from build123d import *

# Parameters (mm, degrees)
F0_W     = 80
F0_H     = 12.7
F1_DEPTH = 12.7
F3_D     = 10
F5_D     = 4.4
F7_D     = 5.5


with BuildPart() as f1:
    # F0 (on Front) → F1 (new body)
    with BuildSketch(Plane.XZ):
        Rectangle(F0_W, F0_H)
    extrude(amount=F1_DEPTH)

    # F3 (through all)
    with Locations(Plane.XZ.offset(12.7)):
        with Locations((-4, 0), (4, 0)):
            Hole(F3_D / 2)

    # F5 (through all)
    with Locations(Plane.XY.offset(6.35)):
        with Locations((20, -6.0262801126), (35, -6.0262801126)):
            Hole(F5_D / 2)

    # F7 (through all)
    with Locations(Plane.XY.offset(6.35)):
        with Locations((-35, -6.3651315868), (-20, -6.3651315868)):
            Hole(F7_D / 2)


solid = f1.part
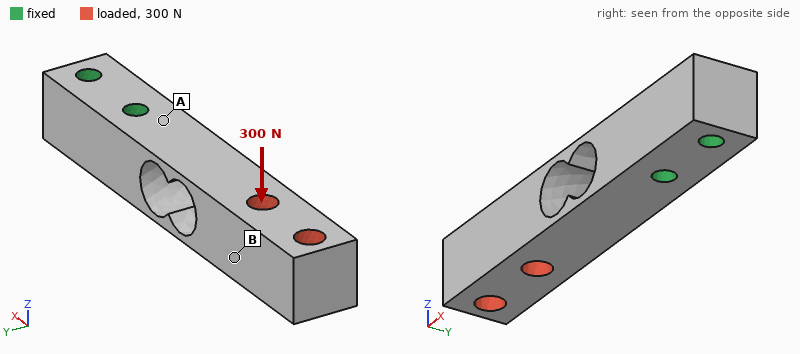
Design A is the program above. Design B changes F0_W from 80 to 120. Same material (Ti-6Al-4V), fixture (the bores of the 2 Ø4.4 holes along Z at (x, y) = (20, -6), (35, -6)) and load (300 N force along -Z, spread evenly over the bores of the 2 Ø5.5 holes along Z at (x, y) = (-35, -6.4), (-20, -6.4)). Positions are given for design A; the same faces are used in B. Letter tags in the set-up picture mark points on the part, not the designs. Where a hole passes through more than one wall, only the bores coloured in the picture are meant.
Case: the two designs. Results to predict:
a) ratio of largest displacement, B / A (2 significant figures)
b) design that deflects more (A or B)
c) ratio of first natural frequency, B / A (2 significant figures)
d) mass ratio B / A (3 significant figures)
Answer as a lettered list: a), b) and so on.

a) 1.2
b) B
c) 0.62
d) 1.64
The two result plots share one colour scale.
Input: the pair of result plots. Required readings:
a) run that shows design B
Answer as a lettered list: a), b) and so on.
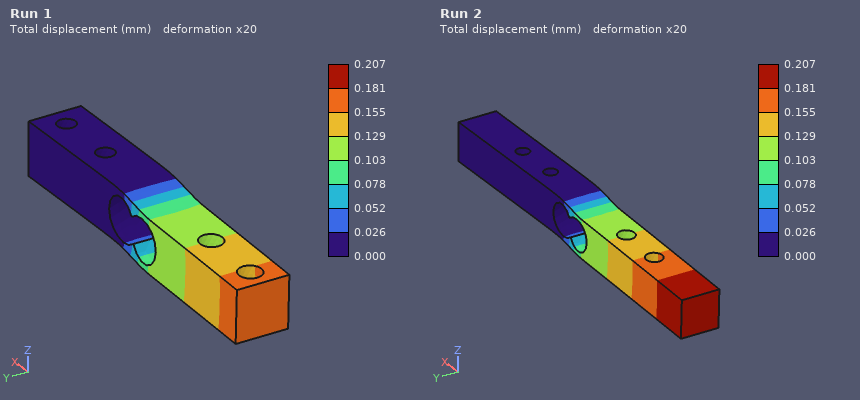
a) Run 2
